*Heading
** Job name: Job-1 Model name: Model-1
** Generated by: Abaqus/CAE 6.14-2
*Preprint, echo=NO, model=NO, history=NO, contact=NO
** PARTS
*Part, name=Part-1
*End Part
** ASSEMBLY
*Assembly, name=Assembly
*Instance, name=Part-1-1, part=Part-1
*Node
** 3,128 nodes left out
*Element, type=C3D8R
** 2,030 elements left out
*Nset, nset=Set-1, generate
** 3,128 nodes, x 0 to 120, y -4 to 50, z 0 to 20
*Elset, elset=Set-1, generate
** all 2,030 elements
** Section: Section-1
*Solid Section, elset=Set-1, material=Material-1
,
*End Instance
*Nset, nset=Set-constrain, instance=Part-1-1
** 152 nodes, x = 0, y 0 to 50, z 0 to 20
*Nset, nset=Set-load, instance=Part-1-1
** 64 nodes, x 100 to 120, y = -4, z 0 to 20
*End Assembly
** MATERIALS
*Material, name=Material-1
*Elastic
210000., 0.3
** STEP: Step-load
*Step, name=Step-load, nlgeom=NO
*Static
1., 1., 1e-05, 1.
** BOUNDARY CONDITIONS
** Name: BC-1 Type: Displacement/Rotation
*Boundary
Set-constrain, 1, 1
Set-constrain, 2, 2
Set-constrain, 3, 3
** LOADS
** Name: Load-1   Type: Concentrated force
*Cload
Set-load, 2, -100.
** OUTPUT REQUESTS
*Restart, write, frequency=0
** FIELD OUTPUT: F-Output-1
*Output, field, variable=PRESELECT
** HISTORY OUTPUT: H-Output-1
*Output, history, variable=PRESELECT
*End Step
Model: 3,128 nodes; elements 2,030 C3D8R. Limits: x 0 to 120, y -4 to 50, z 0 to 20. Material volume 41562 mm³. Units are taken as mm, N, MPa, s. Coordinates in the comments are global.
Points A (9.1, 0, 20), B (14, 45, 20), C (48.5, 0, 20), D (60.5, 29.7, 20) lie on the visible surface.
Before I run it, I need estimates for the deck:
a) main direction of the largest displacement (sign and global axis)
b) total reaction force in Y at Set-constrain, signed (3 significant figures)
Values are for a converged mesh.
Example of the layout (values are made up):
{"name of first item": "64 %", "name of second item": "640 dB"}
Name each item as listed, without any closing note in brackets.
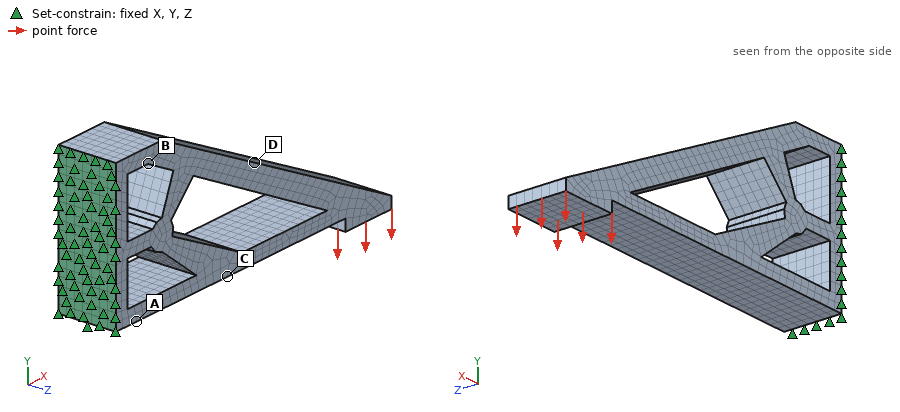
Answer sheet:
{"main direction of the largest displacement": "-Y", "total reaction force in Y at Set-constrain, signed": "6400 N"}
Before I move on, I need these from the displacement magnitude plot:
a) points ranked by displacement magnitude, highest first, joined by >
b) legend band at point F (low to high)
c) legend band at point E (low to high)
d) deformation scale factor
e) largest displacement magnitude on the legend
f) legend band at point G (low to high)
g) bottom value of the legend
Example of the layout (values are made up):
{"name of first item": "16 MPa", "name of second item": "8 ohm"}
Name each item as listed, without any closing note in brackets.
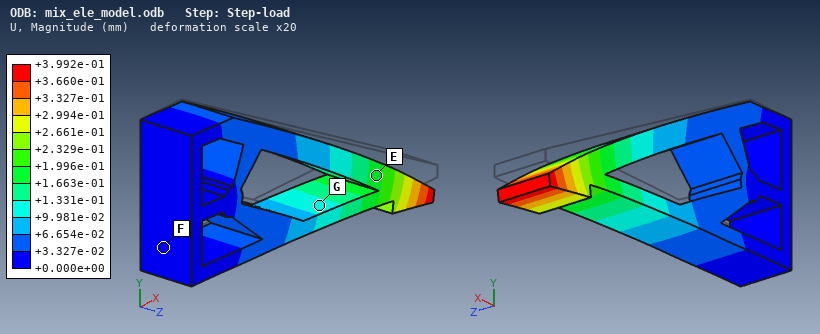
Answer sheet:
{"points ranked by displacement magnitude, highest first, joined by >": "E > G > F", "legend band at point F": "+0.000e+00 to +3.327e-02 mm", "legend band at point E": "+1.663e-01 to +1.996e-01 mm", "deformation scale factor": "20", "largest displacement magnitude on the legend": "+3.992e-01 mm", "legend band at point G": "+9.981e-02 to +1.331e-01 mm", "bottom value of the legend": "+0.000e+00 mm"}
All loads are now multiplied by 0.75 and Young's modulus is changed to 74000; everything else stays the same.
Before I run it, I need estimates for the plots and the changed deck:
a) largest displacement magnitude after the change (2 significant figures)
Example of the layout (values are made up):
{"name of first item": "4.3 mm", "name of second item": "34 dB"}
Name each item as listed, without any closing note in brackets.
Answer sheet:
{"largest displacement magnitude after the change": "0.85 mm"}
